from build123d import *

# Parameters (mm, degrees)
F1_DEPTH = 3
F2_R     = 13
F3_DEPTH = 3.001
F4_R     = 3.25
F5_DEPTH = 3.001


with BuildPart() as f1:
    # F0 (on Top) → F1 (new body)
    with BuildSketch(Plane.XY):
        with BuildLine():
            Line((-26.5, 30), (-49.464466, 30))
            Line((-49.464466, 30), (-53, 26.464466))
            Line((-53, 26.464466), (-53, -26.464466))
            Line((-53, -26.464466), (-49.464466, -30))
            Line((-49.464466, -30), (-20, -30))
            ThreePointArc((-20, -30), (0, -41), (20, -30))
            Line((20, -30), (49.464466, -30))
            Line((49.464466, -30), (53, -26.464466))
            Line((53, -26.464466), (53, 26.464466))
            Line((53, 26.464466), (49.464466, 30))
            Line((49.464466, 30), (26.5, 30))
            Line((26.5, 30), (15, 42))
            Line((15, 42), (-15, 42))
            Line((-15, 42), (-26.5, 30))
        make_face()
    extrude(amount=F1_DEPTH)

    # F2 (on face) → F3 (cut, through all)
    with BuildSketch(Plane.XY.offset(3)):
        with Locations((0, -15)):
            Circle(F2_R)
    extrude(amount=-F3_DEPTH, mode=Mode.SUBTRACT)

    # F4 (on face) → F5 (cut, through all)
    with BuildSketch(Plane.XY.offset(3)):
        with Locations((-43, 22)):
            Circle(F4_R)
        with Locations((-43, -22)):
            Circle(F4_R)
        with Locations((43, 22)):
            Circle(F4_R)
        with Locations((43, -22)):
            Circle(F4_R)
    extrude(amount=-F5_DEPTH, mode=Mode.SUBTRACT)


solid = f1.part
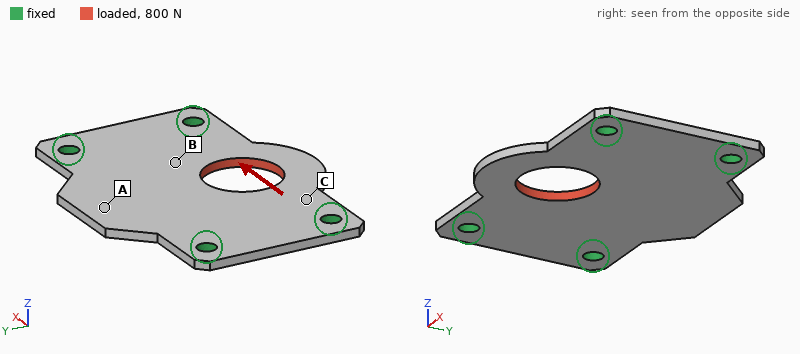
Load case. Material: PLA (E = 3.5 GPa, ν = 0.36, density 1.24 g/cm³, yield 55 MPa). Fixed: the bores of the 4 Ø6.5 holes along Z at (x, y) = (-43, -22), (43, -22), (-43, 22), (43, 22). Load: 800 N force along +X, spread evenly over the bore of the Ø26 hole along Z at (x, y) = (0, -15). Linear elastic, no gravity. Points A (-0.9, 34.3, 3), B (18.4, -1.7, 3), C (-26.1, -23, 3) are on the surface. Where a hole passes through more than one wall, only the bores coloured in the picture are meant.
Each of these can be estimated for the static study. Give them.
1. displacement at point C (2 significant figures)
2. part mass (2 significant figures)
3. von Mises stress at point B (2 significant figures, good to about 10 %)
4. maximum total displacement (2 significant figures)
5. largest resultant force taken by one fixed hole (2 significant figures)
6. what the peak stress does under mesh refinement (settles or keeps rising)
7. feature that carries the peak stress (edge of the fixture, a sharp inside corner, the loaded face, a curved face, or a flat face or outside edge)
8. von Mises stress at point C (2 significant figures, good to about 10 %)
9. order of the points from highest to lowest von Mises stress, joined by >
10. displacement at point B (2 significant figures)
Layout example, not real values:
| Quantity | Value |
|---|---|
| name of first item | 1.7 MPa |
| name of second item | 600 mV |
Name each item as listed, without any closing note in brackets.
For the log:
| Quantity | Value |
|---|---|
| displacement at point C | 23 µm |
| part mass | 24 g |
| von Mises stress at point B | 2.3 MPa |
| maximum total displacement | 59 µm |
| largest resultant force taken by one fixed hole | 270 N |
| what the peak stress does under mesh refinement | keeps rising |
| feature that carries the peak stress | edge of the fixture |
| von Mises stress at point C | 4.7 MPa |
| order of the points from highest to lowest von Mises stress, joined by > | C > B > A |
| displacement at point B | 23 µm |
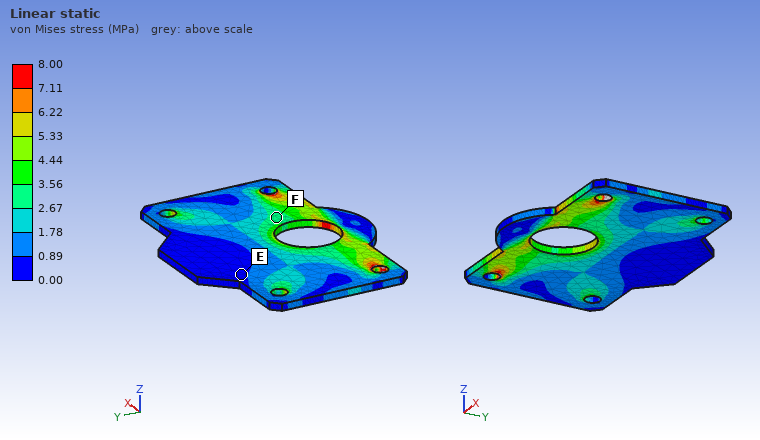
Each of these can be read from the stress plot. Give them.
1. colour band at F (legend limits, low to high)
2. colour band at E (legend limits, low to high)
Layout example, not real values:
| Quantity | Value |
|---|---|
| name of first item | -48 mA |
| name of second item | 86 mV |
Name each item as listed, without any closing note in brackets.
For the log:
| Quantity | Value |
|---|---|
| colour band at F | 2.67 to 3.56 MPa |
| colour band at E | 0.00 to 0.89 MPa |
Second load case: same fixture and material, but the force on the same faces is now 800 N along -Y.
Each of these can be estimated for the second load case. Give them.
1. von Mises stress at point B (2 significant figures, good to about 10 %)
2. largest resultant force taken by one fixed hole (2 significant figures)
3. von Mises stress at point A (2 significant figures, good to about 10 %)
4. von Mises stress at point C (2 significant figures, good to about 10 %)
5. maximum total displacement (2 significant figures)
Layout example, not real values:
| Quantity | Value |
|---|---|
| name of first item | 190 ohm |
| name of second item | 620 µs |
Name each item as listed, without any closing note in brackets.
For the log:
| Quantity | Value |
|---|---|
| von Mises stress at point B | 4.5 MPa |
| largest resultant force taken by one fixed hole | 250 N |
| von Mises stress at point A | 1.6 MPa |
| von Mises stress at point C | 3.5 MPa |
| maximum total displacement | 0.11 mm |
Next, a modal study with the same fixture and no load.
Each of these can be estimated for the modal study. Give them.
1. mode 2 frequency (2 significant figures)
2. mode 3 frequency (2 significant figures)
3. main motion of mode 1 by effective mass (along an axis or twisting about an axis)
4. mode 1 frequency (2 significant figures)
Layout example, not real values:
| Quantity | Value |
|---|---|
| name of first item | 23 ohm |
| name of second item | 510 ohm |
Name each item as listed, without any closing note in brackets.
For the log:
| Quantity | Value |
|---|---|
| mode 2 frequency | 760 Hz |
| mode 3 frequency | 1200 Hz |
| main motion of mode 1 by effective mass | along Z |
| mode 1 frequency | 660 Hz |
